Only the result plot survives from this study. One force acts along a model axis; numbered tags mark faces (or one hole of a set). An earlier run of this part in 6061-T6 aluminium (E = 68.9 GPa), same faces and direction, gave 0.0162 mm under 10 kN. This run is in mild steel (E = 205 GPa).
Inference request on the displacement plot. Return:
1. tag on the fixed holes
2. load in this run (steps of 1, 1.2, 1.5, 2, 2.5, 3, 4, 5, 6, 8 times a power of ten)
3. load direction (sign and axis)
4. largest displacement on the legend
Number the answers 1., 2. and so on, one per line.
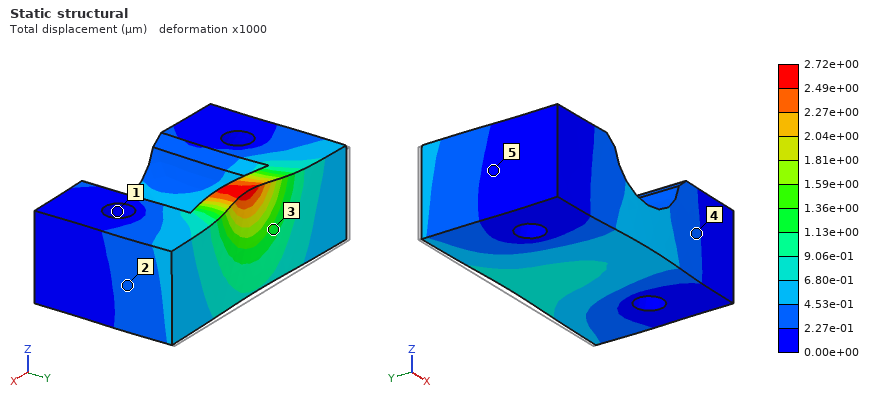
1. 1
2. 5 kN
3. -Y
4. 2.72e+00 µm
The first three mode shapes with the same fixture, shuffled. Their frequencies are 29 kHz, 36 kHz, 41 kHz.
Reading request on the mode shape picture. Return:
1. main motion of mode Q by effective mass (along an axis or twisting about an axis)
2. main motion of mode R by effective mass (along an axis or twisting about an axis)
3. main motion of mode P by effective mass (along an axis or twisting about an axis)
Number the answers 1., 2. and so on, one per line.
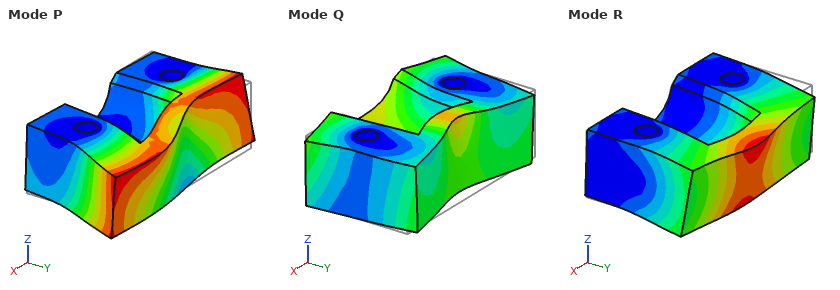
1. along Y
2. along Z
3. along X
